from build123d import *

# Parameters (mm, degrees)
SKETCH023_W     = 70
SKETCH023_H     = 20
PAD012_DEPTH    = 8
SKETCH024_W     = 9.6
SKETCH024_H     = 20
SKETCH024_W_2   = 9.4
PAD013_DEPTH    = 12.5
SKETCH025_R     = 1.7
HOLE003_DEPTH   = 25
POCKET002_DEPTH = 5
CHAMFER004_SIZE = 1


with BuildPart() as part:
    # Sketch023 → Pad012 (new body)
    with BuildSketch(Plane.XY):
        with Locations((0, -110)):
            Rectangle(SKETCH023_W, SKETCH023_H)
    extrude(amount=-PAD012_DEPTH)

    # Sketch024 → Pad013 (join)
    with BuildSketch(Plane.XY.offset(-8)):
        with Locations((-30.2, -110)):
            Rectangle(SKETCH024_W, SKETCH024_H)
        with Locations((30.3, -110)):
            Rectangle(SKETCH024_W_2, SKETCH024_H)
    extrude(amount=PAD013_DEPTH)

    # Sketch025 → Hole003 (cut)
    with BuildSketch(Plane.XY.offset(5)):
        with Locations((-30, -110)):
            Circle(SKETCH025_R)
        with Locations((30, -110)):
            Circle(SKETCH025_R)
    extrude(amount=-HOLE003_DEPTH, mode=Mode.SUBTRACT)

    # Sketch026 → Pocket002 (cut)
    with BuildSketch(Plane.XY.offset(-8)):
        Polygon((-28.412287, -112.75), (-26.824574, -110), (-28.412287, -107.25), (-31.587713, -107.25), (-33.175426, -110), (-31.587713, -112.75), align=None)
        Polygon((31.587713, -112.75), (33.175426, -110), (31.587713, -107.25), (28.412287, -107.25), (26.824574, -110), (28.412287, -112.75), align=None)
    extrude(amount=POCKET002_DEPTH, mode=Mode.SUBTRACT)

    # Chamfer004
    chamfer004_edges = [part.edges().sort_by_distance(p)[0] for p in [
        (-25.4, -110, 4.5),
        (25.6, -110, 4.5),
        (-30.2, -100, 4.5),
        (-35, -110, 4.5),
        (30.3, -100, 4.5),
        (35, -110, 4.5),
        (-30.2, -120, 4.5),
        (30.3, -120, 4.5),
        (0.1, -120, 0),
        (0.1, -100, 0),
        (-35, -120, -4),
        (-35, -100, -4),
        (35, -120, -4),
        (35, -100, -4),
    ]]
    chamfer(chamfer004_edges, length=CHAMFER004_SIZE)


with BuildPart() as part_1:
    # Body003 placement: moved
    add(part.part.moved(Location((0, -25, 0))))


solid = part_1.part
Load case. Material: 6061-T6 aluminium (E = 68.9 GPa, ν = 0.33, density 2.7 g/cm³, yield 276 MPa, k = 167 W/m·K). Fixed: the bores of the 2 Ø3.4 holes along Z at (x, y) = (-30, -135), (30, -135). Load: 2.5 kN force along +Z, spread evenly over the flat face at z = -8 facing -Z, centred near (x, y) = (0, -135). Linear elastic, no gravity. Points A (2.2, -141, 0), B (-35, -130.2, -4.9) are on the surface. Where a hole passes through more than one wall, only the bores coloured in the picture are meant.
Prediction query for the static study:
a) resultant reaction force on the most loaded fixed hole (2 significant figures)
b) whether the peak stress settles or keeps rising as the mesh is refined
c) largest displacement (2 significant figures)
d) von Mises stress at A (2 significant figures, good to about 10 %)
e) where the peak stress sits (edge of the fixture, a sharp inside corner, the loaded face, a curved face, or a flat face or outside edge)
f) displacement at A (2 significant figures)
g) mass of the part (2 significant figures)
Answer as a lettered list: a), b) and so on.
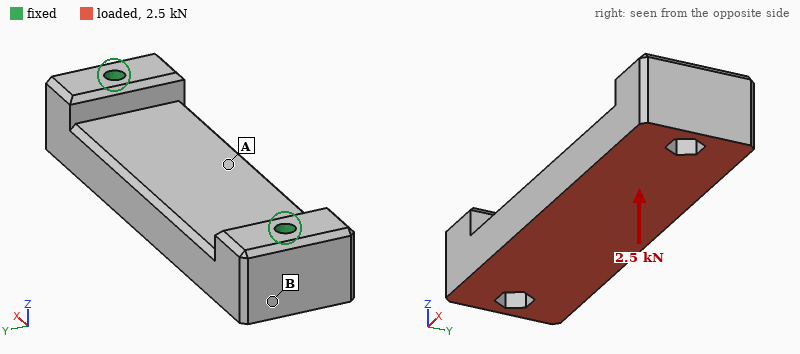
a) 1.6 kN
b) keeps rising
c) 33 µm
d) 24 MPa
e) edge of the fixture
f) 32 µm
g) 33 g
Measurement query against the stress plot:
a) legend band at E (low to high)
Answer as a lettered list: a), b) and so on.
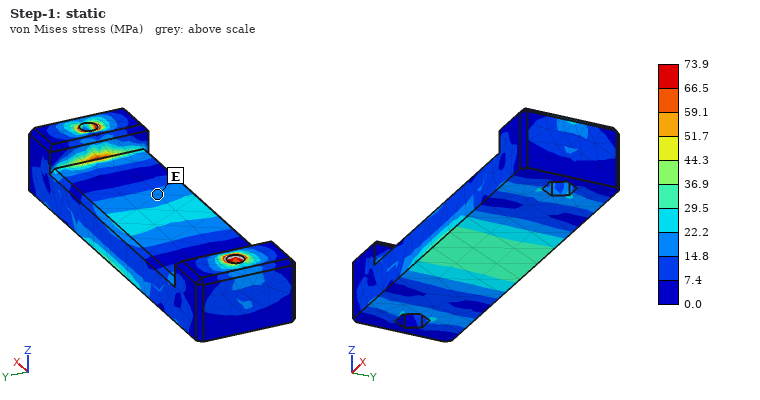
a) 14.8 to 22.2 MPa
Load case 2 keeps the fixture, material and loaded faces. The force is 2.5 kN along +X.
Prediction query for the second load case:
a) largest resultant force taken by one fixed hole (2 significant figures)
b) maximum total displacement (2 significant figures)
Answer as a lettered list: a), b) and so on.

a) 1.3 kN
b) 5.3 µm
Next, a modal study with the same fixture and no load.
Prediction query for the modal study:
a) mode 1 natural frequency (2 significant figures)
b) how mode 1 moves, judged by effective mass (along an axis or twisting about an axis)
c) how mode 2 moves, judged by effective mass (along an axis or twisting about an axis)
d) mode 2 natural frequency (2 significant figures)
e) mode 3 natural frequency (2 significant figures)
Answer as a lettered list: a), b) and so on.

a) 9200 Hz
b) along Z
c) along Y
d) 11 kHz
e) 16 kHz
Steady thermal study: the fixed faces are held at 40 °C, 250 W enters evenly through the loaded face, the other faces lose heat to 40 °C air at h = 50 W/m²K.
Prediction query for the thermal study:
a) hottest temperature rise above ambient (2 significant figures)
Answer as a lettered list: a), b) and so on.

a) 82 K
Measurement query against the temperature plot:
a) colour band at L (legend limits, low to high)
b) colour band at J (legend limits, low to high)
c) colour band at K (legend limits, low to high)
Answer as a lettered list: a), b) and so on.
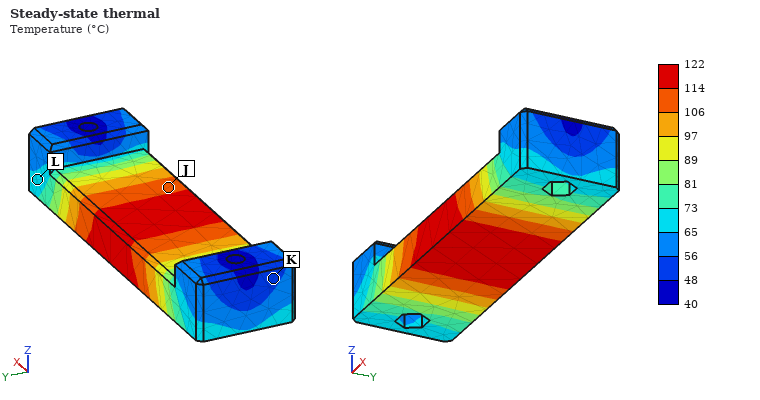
a) 65 to 73 °C
b) 106 to 114 °C
c) 48 to 56 °C
